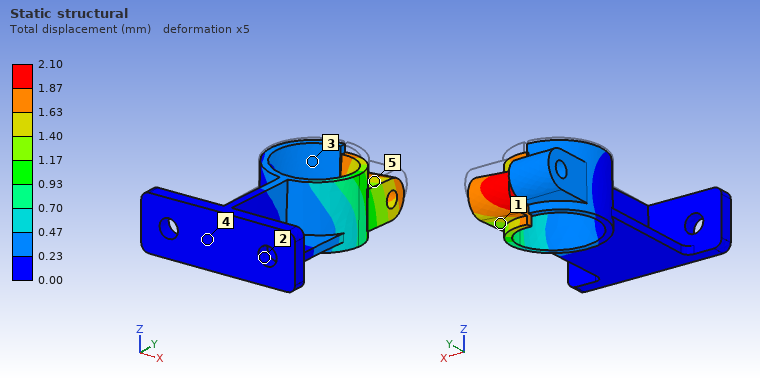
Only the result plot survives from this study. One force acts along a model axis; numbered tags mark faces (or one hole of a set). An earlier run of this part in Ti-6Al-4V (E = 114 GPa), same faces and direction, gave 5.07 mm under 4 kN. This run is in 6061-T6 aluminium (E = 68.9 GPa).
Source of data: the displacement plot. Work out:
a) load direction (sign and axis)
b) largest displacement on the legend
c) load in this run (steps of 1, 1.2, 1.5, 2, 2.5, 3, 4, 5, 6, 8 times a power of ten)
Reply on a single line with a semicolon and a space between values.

-Z; 2.10 mm; 1 kN
